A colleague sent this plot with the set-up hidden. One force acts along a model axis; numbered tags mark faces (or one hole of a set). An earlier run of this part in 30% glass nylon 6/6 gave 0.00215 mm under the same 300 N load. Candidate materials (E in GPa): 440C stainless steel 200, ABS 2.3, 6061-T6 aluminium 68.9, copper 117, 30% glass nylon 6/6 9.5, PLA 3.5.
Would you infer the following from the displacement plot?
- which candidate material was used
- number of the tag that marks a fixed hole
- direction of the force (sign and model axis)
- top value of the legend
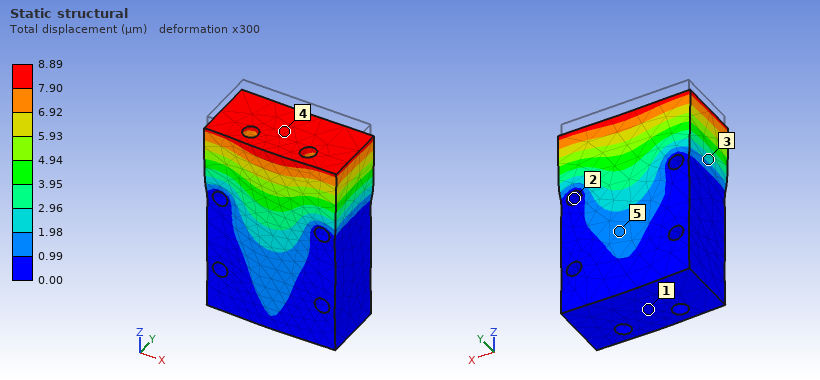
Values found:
ABS
2
-Z
8.89 µm
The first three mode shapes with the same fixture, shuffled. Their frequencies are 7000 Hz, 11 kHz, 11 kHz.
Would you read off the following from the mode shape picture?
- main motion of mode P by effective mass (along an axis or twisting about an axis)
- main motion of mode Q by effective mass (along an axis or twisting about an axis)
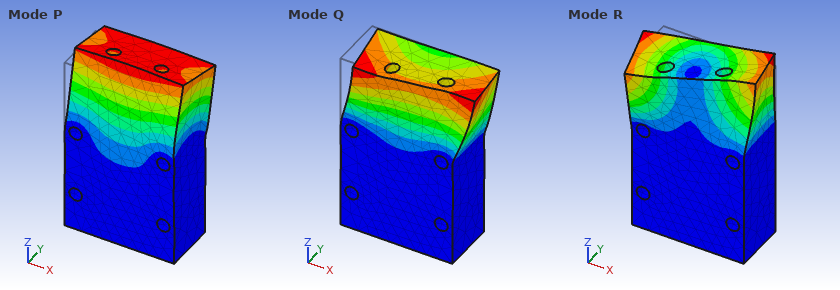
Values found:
along Y
along X
